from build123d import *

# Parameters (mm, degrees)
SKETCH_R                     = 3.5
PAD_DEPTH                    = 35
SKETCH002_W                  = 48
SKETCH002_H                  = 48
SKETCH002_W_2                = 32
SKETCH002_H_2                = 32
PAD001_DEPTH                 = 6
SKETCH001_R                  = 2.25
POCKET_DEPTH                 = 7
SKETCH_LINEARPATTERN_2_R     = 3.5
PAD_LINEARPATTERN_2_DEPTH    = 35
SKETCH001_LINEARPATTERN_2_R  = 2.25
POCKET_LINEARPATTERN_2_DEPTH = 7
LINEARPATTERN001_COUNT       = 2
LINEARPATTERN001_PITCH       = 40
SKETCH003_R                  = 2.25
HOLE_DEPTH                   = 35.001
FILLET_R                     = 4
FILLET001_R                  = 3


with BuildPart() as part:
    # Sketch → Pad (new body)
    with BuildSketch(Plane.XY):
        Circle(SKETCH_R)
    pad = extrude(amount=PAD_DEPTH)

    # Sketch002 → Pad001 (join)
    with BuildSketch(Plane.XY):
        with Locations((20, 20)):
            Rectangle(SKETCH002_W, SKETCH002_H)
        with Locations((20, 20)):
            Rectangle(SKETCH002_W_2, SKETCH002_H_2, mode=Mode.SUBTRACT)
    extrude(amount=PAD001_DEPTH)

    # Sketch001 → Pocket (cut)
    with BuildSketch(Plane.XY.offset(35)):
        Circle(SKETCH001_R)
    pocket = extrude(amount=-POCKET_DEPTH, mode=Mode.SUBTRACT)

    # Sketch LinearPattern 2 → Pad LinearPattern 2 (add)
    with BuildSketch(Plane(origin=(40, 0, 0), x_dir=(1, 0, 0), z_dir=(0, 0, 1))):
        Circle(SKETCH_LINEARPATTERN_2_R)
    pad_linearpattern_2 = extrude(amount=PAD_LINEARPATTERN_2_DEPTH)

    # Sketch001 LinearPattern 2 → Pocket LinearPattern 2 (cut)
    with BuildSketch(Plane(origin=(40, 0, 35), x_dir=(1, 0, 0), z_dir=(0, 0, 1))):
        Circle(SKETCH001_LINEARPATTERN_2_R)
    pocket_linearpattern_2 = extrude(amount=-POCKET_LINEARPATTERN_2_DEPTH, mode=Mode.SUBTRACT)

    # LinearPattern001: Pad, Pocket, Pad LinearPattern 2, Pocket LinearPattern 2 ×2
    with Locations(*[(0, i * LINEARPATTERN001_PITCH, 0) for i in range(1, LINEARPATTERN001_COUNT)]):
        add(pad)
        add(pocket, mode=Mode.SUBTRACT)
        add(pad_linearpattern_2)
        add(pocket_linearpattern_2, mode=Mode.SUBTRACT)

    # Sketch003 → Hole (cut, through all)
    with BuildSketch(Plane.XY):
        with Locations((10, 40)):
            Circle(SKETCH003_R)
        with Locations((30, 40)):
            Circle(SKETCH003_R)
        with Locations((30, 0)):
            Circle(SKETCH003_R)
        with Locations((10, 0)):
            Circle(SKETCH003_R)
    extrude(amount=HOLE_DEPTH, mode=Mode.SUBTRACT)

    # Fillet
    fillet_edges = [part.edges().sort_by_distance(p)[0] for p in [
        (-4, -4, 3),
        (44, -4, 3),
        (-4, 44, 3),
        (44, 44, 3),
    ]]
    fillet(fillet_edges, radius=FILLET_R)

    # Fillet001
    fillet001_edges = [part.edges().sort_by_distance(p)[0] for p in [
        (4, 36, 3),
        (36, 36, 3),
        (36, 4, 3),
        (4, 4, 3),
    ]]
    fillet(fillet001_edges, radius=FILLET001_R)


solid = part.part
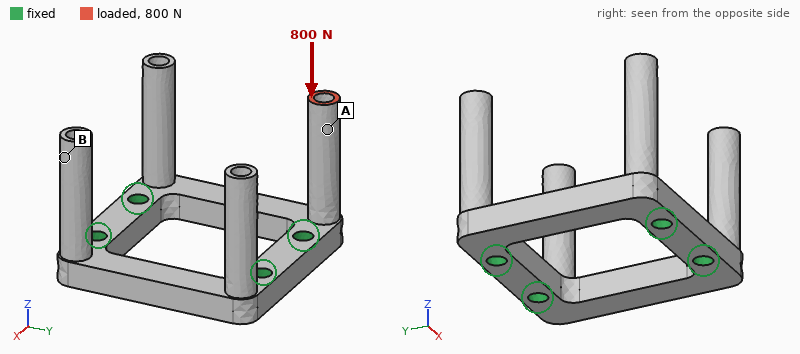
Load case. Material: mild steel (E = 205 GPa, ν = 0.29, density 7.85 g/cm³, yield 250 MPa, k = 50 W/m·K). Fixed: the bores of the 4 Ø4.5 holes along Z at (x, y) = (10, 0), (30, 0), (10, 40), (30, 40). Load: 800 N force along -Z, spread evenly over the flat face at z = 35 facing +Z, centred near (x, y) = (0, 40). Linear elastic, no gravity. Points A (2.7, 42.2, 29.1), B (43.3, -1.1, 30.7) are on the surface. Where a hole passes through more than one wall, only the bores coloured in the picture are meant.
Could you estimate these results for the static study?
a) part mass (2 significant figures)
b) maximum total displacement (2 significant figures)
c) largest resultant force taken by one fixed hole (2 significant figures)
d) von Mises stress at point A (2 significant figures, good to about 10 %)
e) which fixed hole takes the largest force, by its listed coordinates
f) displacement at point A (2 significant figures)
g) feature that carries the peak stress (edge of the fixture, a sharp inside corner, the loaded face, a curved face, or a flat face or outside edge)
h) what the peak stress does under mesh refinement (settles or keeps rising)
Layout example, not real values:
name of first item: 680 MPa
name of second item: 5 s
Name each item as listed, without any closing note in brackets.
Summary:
part mass: 89 g
maximum total displacement: 32 µm
largest resultant force taken by one fixed hole: 800 N
von Mises stress at point A: 32 MPa
which fixed hole takes the largest force, by its listed coordinates: (10, 40)
displacement at point A: 25 µm
feature that carries the peak stress: edge of the fixture
what the peak stress does under mesh refinement: keeps rising
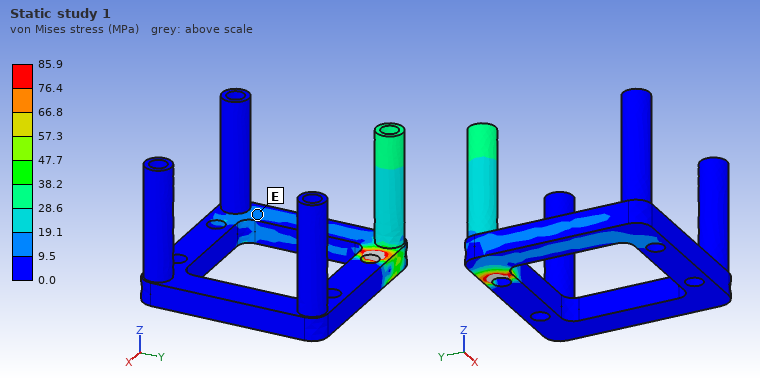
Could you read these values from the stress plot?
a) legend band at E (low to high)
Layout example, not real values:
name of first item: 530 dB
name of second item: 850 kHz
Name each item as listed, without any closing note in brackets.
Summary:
legend band at E: 9.5 to 19.1 MPa
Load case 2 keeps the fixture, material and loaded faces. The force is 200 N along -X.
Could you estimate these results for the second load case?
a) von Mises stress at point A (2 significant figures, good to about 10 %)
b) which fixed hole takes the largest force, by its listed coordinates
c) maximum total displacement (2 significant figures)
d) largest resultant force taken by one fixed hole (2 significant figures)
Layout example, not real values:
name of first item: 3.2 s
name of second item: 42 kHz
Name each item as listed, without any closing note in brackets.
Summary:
von Mises stress at point A: 35 MPa
which fixed hole takes the largest force, by its listed coordinates: (10, 40)
maximum total displacement: 0.13 mm
largest resultant force taken by one fixed hole: 200 N
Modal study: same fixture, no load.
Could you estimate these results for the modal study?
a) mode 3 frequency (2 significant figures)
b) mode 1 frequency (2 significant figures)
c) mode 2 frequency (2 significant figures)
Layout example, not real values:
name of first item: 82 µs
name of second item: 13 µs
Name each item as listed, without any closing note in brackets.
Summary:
mode 3 frequency: 4600 Hz
mode 1 frequency: 4300 Hz
mode 2 frequency: 4400 Hz
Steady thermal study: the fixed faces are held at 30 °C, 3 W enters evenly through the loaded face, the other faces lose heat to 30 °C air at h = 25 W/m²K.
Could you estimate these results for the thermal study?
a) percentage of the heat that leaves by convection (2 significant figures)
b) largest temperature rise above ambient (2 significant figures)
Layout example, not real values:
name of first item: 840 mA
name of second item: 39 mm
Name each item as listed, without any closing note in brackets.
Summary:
percentage of the heat that leaves by convection: 22 %
largest temperature rise above ambient: 55 K
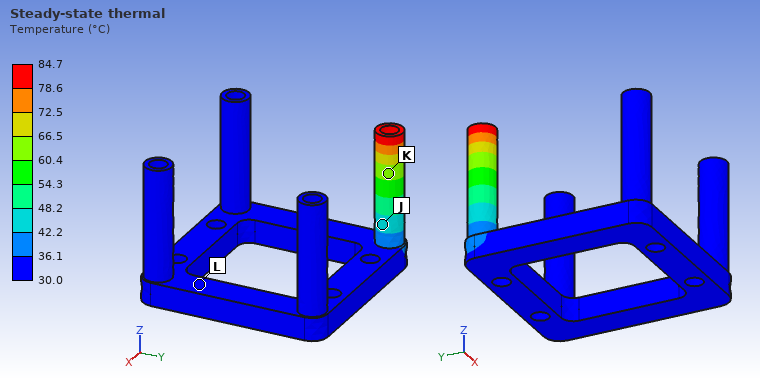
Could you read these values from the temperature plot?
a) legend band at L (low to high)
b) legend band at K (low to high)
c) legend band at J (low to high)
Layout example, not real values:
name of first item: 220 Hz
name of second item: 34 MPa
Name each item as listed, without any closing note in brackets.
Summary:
legend band at L: 30.0 to 36.1 °C
legend band at K: 60.4 to 66.5 °C
legend band at J: 42.2 to 48.2 °C
